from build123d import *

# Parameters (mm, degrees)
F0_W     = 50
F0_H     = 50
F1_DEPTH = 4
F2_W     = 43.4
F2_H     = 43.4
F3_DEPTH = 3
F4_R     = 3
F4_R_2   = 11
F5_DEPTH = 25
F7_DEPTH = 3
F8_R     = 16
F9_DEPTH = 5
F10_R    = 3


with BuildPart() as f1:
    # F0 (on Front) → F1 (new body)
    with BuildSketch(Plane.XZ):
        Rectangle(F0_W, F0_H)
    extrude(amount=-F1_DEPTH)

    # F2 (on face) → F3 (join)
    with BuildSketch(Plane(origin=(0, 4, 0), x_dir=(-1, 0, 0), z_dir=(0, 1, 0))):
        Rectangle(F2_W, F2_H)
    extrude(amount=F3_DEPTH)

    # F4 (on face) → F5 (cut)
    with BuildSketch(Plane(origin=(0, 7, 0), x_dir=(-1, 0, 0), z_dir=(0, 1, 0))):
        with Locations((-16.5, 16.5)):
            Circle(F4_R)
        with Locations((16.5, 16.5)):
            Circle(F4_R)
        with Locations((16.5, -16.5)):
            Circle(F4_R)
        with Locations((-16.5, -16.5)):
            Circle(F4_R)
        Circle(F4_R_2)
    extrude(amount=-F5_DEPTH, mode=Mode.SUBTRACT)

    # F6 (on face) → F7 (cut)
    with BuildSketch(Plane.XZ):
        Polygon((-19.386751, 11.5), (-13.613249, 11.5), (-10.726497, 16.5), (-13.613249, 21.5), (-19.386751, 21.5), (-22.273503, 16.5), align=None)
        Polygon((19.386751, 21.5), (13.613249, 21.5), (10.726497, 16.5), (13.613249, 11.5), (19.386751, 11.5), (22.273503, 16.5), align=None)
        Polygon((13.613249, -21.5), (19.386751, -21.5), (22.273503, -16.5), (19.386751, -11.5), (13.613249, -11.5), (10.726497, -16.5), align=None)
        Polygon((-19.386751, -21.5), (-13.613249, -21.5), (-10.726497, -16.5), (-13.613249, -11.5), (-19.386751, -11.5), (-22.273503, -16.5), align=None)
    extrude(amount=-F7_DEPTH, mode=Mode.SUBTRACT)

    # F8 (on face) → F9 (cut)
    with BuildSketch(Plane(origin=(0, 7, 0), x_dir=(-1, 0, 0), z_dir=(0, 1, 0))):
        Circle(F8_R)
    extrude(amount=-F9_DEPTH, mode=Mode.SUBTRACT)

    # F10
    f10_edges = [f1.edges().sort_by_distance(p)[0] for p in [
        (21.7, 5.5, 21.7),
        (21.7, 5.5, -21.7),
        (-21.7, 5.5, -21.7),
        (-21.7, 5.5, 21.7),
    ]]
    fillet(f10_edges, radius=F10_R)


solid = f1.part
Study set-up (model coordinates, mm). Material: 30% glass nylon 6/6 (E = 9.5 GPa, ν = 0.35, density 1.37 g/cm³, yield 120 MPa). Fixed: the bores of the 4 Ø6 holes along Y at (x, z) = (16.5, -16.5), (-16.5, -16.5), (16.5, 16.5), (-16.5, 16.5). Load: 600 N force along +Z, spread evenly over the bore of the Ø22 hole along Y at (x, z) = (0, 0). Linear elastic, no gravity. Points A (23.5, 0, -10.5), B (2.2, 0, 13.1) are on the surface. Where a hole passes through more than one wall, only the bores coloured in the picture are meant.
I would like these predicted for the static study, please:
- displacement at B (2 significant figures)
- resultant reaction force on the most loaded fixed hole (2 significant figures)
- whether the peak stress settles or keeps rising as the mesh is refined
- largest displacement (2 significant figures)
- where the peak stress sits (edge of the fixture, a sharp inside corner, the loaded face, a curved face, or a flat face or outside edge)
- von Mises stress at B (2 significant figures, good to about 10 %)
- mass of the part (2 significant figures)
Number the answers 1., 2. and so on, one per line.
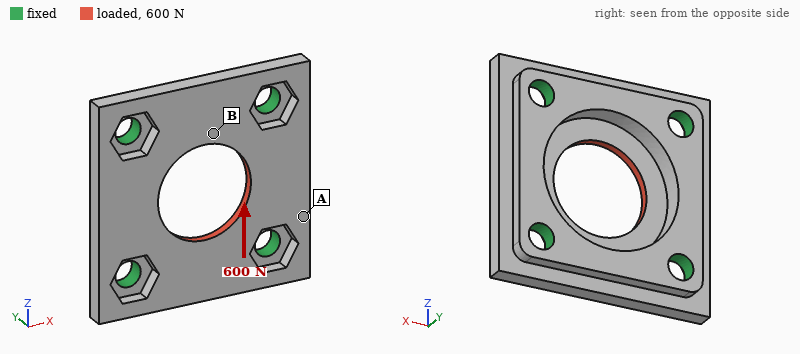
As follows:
1. 14 µm
2. 150 N
3. keeps rising
4. 17 µm
5. edge of the fixture
6. 4.2 MPa
7. 13 g
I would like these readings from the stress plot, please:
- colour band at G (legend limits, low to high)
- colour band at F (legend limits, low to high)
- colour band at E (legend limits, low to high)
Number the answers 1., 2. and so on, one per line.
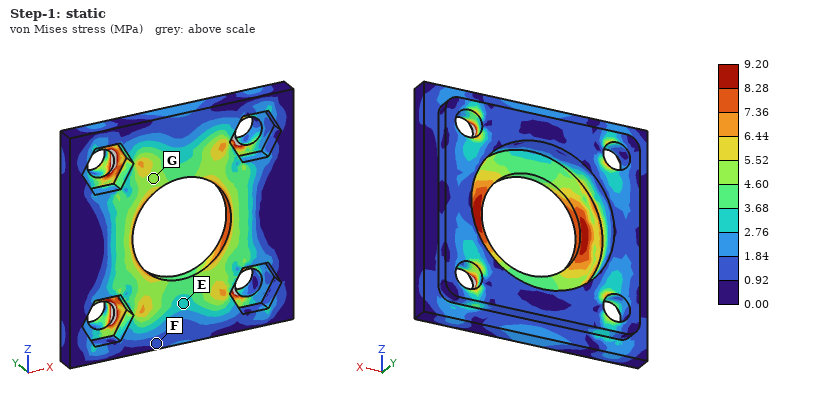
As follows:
1. 4.60 to 5.52 MPa
2. 0.92 to 1.84 MPa
3. 2.76 to 3.68 MPa
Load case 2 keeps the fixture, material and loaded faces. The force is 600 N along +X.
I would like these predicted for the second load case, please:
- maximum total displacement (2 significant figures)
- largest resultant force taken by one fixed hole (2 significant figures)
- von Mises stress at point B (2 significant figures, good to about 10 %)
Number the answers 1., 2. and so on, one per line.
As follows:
1. 17 µm
2. 150 N
3. 4.5 MPa
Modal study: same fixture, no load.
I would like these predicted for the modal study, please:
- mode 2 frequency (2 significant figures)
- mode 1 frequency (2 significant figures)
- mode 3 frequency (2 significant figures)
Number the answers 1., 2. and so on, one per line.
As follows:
1. 13 kHz
2. 12 kHz
3. 13 kHz
